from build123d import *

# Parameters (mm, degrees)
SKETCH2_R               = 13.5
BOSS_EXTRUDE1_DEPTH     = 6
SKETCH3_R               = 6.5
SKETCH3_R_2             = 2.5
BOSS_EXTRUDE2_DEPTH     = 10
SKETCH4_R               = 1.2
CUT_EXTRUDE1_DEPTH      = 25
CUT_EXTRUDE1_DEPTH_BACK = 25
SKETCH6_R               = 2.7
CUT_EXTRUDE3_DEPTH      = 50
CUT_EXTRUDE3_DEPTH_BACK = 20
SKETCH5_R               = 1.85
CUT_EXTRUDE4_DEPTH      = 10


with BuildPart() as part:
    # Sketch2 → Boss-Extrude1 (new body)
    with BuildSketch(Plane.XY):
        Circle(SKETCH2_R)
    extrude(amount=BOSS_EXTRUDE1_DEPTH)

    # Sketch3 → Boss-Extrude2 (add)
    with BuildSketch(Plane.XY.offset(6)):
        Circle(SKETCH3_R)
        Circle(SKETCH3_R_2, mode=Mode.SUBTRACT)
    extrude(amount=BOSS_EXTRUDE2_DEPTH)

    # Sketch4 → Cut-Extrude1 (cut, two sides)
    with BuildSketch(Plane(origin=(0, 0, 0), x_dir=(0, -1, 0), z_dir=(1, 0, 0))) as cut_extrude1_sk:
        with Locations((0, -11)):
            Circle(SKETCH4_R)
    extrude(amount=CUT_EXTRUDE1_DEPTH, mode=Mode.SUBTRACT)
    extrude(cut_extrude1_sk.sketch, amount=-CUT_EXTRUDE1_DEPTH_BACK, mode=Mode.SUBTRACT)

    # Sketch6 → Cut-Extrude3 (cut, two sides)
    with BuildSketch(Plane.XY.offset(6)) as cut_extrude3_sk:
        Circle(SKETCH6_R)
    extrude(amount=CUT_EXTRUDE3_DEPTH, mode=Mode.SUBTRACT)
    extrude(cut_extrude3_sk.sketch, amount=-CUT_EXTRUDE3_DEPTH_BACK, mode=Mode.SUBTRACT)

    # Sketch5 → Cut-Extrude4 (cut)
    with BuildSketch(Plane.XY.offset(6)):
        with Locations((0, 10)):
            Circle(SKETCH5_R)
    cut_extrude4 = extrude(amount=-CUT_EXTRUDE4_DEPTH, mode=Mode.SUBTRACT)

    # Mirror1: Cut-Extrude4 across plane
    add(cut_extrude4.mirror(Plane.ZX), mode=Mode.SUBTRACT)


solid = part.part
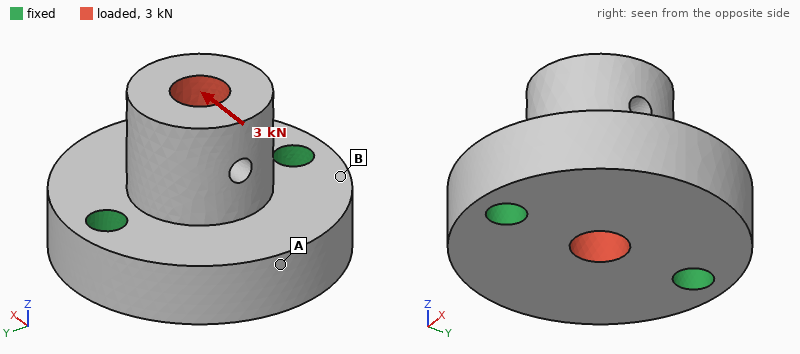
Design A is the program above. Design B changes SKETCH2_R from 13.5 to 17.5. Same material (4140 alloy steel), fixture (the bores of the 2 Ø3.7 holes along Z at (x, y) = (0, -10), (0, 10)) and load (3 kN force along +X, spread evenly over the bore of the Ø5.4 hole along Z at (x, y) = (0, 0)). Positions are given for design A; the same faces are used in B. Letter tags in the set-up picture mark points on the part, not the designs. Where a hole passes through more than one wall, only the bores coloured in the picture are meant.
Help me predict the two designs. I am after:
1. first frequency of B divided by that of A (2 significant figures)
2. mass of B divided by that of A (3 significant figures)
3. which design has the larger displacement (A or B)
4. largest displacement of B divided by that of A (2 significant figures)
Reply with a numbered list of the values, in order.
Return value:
1. 0.78
2. 1.55
3. A
4. 0.90
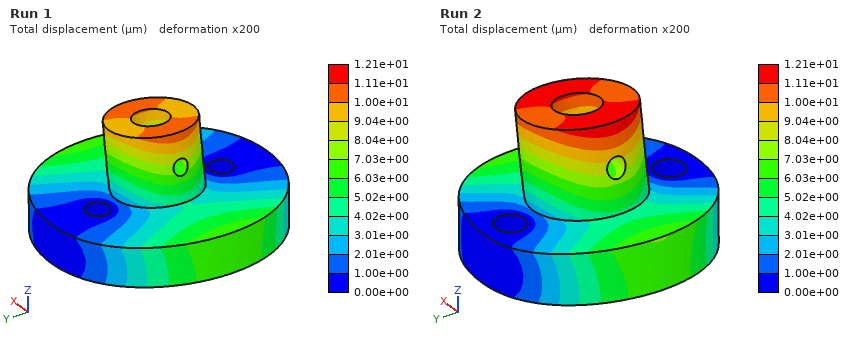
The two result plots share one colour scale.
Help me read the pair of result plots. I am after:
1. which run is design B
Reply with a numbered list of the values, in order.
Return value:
1. Run 1
